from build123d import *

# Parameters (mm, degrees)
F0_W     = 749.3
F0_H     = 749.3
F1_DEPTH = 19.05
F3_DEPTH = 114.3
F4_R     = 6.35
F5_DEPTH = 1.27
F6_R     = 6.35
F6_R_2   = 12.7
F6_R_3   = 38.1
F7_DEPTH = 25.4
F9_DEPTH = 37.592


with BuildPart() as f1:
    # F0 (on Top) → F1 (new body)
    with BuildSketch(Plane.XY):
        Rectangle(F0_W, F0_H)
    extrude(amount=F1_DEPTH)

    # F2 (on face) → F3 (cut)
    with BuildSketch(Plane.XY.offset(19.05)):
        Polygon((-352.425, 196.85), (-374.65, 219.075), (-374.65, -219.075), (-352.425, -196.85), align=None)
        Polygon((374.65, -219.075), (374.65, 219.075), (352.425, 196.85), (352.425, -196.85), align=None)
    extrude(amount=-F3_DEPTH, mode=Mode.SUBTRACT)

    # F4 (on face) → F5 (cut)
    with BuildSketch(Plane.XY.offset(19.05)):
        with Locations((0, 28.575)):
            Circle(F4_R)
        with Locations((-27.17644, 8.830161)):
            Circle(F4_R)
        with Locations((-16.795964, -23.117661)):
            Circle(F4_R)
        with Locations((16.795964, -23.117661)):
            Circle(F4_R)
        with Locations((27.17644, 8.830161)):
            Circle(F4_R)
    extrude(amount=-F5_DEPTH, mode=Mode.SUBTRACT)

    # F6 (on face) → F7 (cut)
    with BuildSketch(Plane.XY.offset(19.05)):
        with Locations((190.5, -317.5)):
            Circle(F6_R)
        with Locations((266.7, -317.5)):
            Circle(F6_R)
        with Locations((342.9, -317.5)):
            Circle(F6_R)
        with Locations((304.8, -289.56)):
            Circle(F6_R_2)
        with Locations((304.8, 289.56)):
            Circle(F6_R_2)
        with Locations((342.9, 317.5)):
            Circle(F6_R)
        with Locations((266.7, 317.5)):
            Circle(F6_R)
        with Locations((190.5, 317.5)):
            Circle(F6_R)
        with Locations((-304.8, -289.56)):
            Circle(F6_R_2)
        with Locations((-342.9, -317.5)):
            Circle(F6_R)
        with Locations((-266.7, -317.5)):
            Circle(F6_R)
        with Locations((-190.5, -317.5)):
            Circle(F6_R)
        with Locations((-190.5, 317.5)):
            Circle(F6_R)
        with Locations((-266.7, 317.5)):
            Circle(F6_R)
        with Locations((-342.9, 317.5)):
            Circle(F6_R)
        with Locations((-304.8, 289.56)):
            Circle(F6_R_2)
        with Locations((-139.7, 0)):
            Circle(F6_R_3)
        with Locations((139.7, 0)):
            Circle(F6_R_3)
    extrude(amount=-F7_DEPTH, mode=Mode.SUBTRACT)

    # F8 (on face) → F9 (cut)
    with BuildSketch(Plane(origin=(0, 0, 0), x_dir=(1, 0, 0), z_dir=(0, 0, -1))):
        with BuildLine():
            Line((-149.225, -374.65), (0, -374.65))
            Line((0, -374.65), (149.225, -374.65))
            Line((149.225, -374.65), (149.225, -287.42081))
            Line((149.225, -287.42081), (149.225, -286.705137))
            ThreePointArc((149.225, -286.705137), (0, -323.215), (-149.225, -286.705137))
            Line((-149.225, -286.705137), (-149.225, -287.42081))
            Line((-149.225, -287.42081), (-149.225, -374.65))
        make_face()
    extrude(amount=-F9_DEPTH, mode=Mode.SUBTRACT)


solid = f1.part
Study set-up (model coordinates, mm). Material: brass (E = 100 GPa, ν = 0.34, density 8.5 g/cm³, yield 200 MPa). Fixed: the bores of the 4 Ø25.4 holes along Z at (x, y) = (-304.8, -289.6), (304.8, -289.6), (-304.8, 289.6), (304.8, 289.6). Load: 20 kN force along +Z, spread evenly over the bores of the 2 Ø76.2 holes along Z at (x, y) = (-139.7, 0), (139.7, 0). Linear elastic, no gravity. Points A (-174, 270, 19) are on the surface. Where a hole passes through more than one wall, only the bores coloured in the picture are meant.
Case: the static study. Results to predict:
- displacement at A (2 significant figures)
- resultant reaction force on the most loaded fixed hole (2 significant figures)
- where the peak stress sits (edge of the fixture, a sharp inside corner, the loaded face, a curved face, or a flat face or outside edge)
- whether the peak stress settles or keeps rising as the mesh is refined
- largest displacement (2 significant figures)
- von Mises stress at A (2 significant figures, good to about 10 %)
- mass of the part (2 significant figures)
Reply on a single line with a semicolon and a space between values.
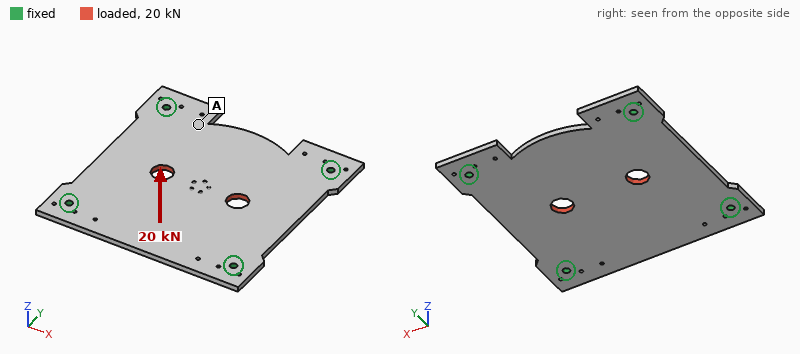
0.27 mm; 5.0 kN; edge of the fixture; keeps rising; 1.3 mm; 18 MPa; 83 kg
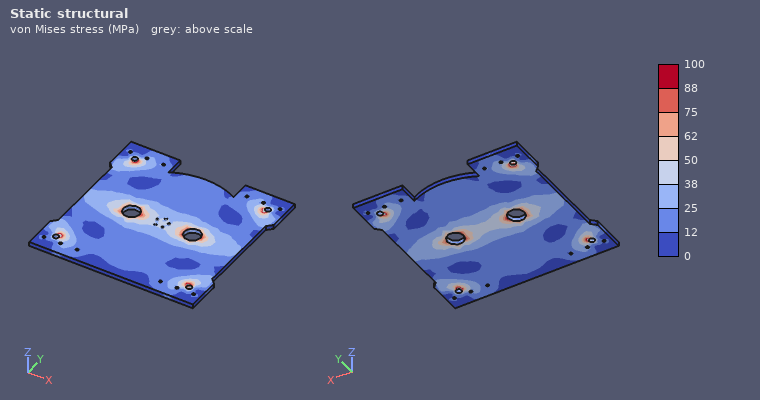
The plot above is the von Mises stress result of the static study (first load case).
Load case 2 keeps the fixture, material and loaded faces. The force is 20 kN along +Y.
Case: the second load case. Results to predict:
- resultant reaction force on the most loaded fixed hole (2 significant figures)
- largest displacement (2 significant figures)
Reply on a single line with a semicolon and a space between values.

5.5 kN; 7.8 µm
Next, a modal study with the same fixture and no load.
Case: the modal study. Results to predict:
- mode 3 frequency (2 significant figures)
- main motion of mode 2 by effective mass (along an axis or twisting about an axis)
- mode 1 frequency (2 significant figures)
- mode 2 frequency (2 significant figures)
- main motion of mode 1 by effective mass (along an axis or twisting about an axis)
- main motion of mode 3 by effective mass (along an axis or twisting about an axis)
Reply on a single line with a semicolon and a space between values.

220 Hz; twisting about X; 120 Hz; 200 Hz; along Z; twisting about Y
